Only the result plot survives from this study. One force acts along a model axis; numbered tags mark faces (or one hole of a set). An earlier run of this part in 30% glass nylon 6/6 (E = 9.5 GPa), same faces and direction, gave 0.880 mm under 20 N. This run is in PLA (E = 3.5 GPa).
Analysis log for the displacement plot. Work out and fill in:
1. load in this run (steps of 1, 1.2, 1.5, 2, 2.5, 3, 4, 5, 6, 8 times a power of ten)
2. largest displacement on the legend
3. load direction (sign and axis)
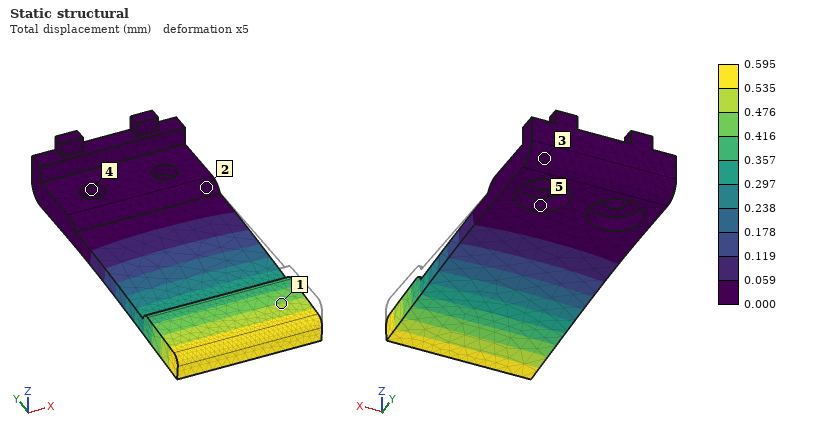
5 N
0.595 mm
-Z
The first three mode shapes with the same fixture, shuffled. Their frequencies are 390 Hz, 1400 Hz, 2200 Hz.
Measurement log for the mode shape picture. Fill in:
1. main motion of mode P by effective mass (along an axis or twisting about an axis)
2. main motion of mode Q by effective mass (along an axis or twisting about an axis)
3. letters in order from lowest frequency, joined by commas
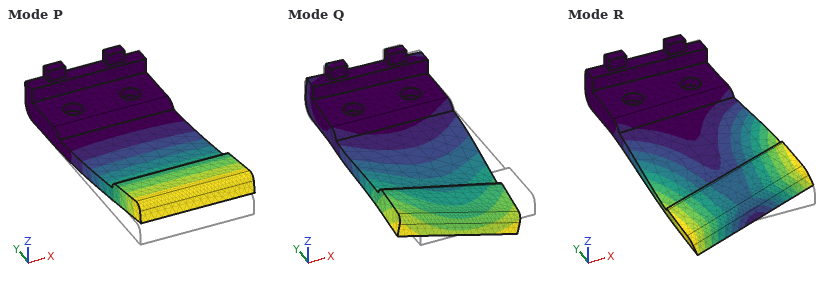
along Z
along X
P, R, Q
